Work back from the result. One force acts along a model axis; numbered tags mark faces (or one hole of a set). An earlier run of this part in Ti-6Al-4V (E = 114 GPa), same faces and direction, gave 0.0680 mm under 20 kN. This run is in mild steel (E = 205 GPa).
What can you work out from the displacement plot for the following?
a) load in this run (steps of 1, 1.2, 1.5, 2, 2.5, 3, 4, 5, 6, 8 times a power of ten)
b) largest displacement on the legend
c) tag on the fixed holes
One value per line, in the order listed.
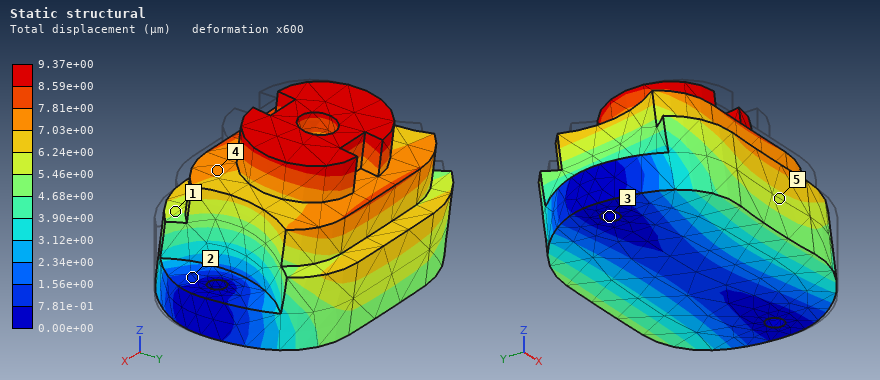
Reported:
5 kN
9.37e+00 µm
3
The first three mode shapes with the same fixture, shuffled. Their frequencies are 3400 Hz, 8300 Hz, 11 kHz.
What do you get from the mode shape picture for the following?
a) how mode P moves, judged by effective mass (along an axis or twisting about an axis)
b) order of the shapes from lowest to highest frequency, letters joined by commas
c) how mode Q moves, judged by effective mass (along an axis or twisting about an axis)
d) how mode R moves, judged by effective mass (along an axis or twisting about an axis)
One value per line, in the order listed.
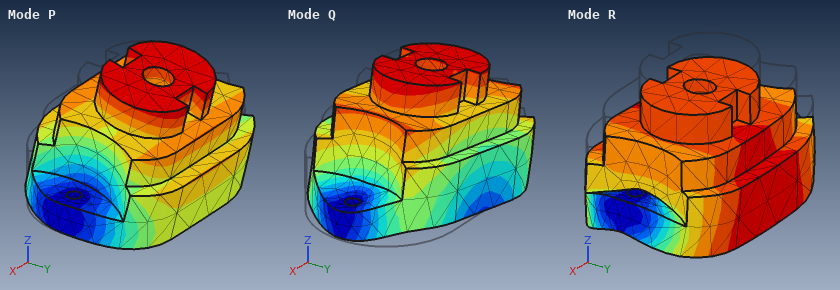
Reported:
along Y
P, R, Q
along X
along Z
